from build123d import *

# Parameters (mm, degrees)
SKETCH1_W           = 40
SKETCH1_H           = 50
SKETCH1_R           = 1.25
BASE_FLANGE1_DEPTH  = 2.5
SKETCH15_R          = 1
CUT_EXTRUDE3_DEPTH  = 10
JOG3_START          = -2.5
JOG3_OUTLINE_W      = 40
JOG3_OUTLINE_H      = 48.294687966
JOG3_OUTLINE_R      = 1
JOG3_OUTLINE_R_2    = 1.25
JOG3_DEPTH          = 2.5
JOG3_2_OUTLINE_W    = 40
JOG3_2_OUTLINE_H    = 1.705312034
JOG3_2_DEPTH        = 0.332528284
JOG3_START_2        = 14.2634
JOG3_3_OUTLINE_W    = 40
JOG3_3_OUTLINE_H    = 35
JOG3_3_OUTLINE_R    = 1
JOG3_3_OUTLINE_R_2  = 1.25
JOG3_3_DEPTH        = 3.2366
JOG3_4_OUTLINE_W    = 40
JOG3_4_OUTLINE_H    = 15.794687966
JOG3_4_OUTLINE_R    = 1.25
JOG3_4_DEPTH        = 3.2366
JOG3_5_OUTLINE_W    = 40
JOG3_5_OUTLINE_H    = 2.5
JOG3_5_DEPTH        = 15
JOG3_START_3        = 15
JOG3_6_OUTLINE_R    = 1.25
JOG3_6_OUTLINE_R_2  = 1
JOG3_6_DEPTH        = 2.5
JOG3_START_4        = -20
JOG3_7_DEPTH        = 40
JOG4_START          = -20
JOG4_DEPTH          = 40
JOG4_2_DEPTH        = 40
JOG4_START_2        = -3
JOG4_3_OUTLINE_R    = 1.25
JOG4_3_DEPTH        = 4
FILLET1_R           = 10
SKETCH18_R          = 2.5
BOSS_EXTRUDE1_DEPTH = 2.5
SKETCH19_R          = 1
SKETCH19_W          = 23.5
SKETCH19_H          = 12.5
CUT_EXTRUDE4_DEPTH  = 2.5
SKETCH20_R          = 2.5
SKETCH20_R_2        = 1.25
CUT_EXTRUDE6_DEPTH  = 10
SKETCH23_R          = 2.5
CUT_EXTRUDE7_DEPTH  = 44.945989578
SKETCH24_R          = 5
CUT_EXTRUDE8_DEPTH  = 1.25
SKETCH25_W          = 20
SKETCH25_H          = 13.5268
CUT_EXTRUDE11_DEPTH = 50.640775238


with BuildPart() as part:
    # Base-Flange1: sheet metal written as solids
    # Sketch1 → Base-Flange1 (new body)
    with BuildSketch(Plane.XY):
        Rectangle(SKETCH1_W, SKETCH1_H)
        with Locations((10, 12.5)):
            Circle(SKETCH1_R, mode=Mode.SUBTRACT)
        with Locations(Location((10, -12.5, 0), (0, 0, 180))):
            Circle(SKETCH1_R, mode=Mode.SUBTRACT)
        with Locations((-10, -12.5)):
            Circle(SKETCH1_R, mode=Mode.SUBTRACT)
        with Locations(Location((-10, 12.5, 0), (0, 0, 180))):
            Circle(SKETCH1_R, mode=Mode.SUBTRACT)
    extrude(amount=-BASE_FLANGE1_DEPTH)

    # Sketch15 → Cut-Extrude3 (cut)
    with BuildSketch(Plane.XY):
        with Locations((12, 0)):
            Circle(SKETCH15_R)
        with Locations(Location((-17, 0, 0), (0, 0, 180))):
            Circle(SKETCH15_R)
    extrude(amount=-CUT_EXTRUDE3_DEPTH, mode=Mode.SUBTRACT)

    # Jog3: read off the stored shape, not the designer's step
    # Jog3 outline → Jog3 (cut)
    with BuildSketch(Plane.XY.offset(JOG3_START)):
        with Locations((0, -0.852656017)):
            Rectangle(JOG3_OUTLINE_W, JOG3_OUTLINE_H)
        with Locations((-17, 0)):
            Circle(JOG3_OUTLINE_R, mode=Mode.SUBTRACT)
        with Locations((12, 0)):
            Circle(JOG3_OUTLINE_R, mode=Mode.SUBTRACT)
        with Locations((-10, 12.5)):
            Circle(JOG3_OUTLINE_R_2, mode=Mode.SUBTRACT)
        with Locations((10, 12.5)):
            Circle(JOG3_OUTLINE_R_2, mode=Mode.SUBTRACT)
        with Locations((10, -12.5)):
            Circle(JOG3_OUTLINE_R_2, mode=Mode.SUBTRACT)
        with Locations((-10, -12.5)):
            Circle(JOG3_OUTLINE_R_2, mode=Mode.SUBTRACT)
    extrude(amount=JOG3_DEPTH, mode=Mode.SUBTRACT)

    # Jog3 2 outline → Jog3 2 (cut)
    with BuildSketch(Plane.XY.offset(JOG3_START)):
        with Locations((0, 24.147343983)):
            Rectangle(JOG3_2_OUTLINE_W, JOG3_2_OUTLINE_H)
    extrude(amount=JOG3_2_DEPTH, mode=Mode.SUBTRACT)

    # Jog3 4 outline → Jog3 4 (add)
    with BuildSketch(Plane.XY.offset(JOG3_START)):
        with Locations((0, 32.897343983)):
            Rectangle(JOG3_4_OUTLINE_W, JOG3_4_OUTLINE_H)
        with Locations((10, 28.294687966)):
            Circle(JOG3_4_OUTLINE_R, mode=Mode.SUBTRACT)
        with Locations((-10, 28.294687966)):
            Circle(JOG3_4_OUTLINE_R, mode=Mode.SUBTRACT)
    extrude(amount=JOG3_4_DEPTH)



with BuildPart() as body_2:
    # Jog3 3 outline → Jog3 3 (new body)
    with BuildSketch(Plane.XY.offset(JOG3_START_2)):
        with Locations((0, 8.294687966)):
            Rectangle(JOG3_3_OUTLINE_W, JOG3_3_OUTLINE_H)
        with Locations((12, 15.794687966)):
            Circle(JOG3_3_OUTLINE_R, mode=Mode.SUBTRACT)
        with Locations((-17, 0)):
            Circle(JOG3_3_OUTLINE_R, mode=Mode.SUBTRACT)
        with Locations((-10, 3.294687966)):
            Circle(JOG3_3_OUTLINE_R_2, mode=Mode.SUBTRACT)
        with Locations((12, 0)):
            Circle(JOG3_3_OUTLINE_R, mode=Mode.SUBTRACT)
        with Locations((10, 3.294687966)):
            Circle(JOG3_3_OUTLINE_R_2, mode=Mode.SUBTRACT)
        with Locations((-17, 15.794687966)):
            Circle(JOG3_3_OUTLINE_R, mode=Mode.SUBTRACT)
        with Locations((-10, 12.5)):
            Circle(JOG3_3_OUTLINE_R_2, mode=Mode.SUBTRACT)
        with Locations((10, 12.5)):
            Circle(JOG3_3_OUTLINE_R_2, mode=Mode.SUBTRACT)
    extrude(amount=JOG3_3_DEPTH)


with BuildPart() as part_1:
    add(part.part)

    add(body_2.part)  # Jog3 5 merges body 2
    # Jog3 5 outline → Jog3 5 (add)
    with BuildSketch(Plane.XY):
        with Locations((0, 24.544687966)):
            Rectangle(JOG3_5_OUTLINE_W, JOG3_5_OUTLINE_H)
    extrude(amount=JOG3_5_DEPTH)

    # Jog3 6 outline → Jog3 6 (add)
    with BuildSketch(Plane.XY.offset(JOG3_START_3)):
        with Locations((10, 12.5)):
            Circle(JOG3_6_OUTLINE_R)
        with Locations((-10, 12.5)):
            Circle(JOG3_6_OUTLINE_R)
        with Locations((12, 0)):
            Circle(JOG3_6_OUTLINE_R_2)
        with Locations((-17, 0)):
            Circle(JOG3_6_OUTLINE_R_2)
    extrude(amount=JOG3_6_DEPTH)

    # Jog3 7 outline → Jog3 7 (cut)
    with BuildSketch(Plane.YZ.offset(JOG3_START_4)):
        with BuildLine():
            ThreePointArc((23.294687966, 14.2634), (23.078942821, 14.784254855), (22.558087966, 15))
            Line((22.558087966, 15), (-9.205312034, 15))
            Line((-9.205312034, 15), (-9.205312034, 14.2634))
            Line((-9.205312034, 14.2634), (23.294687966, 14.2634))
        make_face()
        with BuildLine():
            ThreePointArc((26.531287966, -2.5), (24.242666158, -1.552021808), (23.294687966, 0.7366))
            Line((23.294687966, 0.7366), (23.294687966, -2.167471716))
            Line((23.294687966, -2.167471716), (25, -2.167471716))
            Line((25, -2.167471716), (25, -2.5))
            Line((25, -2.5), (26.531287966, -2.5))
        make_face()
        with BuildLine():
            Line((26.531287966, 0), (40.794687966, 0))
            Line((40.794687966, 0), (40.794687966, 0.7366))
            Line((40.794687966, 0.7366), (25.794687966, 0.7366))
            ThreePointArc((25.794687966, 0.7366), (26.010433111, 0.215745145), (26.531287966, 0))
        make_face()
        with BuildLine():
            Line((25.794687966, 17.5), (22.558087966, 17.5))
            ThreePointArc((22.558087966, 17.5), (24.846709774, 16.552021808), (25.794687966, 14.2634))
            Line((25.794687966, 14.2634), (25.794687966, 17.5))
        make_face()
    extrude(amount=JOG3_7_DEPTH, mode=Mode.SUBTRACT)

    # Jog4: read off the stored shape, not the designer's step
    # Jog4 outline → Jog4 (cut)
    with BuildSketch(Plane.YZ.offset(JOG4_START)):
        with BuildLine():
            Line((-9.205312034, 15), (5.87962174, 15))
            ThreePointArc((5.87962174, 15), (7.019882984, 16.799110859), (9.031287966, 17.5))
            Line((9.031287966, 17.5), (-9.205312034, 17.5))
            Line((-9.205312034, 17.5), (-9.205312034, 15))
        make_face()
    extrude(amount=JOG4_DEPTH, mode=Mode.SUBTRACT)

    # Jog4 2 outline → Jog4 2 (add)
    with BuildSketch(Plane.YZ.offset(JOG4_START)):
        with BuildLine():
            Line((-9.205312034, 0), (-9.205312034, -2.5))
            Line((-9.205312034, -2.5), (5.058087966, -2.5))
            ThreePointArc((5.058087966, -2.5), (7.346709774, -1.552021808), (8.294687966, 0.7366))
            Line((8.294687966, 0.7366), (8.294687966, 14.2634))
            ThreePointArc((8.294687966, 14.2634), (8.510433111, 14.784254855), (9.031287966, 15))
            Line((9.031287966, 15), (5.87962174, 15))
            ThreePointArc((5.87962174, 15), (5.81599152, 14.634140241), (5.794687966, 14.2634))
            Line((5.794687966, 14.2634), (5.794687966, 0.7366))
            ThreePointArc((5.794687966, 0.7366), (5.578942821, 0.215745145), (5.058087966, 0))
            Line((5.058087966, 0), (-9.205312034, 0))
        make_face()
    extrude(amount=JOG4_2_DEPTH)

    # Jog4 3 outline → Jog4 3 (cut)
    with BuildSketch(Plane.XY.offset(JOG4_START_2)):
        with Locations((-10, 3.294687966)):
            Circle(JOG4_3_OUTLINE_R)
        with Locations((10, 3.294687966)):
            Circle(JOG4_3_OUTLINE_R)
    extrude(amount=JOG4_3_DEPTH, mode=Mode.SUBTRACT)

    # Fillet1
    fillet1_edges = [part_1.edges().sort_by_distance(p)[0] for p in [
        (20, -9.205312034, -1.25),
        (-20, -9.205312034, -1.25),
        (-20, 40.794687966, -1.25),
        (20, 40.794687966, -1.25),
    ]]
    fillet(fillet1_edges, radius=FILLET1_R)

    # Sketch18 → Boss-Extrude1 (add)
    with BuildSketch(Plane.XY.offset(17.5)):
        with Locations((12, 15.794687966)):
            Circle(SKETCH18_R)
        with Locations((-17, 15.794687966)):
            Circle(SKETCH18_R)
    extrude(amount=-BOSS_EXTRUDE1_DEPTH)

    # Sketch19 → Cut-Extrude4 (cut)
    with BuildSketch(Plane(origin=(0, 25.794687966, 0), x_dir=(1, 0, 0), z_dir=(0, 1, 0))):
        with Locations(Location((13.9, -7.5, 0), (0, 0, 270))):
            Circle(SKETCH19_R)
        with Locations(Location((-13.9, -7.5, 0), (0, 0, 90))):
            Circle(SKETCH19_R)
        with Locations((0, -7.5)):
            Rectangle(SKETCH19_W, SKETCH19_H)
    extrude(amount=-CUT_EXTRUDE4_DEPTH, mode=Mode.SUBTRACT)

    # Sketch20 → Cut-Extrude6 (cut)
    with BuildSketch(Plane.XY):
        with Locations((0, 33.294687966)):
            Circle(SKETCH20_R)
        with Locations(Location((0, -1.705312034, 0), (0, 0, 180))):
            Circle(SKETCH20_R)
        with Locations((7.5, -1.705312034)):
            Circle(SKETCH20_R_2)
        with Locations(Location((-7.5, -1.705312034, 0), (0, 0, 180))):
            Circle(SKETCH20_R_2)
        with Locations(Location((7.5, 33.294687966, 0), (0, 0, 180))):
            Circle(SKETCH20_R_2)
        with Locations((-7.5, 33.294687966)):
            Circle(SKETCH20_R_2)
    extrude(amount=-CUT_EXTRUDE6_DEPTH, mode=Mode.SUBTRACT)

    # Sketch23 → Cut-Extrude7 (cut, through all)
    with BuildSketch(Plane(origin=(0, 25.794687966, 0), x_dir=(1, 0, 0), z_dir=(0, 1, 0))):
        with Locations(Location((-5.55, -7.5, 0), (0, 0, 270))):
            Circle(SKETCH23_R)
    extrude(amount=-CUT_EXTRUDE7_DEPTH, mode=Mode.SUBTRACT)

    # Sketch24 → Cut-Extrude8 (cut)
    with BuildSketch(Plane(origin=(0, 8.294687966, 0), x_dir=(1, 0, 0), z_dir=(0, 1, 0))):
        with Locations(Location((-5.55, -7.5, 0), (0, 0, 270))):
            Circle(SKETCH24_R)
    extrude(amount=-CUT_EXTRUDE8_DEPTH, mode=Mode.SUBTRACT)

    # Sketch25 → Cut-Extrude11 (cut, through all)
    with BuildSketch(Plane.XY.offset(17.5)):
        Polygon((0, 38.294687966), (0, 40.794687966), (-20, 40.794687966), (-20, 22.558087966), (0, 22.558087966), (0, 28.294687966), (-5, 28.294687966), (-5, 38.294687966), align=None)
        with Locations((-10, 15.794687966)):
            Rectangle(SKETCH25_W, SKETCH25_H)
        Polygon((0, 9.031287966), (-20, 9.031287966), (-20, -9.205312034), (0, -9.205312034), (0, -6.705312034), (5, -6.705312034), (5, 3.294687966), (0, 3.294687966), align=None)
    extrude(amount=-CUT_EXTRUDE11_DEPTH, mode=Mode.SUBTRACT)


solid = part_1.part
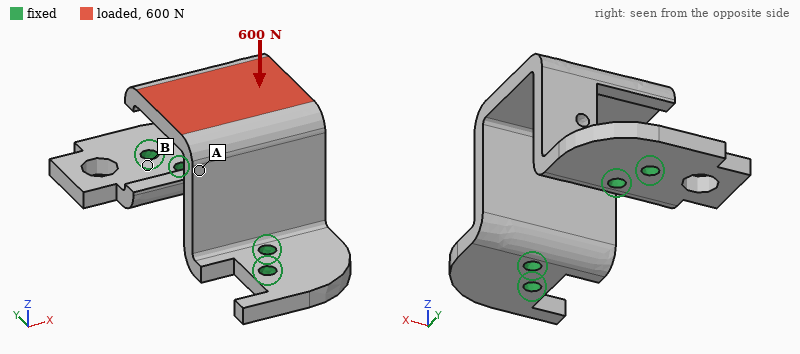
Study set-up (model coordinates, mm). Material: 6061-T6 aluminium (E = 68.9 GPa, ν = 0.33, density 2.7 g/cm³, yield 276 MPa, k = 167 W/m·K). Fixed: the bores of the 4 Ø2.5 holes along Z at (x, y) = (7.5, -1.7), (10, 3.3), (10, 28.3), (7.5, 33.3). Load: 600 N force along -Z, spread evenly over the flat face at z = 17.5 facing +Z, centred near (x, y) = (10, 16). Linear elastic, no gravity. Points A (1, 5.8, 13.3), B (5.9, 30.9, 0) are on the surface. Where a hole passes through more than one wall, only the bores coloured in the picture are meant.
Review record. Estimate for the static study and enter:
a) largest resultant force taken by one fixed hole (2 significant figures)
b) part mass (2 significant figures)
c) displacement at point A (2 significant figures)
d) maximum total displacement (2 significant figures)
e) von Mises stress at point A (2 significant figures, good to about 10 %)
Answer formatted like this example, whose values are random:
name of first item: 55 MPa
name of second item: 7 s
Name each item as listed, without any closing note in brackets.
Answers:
largest resultant force taken by one fixed hole: 330 N
part mass: 9.4 g
displacement at point A: 34 µm
maximum total displacement: 85 µm
von Mises stress at point A: 29 MPa
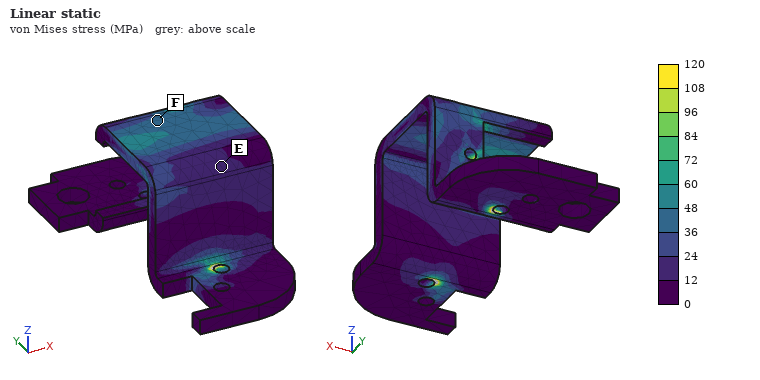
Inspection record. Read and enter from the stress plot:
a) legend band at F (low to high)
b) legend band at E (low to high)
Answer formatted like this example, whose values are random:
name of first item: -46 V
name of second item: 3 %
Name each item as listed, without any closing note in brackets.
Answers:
legend band at F: 36 to 48 MPa
legend band at E: 12 to 24 MPa
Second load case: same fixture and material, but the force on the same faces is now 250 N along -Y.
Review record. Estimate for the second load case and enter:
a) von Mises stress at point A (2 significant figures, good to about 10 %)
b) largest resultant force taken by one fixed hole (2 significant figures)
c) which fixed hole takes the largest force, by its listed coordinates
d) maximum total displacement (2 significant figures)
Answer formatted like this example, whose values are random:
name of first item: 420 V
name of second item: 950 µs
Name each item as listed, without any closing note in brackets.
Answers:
von Mises stress at point A: 37 MPa
largest resultant force taken by one fixed hole: 180 N
which fixed hole takes the largest force, by its listed coordinates: (10, 28.3)
maximum total displacement: 99 µm
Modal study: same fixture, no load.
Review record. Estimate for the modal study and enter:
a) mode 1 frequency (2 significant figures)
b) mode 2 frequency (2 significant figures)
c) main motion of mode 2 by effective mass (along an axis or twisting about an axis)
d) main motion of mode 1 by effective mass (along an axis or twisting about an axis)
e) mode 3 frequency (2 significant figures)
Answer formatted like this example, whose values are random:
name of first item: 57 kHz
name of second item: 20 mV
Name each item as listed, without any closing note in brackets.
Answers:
mode 1 frequency: 4100 Hz
mode 2 frequency: 4800 Hz
main motion of mode 2 by effective mass: along Y
main motion of mode 1 by effective mass: along X
mode 3 frequency: 7300 Hz
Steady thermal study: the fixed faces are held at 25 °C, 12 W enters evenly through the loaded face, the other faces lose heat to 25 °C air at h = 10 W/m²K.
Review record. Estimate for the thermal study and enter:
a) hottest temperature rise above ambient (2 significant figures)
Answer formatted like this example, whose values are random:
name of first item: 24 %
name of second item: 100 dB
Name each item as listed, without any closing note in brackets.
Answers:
hottest temperature rise above ambient: 29 K
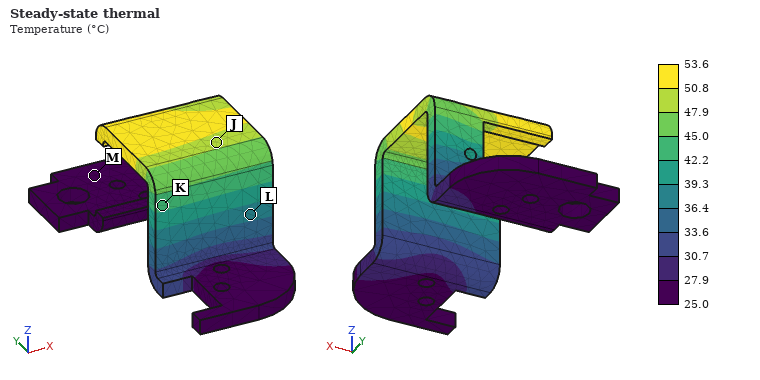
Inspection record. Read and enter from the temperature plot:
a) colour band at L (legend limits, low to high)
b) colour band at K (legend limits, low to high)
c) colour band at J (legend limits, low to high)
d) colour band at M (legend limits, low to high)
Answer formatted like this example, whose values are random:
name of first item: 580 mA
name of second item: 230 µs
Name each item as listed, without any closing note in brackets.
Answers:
colour band at L: 36.4 to 39.3 °C
colour band at K: 42.2 to 45.0 °C
colour band at J: 47.9 to 50.8 °C
colour band at M: 25.0 to 27.9 °C
